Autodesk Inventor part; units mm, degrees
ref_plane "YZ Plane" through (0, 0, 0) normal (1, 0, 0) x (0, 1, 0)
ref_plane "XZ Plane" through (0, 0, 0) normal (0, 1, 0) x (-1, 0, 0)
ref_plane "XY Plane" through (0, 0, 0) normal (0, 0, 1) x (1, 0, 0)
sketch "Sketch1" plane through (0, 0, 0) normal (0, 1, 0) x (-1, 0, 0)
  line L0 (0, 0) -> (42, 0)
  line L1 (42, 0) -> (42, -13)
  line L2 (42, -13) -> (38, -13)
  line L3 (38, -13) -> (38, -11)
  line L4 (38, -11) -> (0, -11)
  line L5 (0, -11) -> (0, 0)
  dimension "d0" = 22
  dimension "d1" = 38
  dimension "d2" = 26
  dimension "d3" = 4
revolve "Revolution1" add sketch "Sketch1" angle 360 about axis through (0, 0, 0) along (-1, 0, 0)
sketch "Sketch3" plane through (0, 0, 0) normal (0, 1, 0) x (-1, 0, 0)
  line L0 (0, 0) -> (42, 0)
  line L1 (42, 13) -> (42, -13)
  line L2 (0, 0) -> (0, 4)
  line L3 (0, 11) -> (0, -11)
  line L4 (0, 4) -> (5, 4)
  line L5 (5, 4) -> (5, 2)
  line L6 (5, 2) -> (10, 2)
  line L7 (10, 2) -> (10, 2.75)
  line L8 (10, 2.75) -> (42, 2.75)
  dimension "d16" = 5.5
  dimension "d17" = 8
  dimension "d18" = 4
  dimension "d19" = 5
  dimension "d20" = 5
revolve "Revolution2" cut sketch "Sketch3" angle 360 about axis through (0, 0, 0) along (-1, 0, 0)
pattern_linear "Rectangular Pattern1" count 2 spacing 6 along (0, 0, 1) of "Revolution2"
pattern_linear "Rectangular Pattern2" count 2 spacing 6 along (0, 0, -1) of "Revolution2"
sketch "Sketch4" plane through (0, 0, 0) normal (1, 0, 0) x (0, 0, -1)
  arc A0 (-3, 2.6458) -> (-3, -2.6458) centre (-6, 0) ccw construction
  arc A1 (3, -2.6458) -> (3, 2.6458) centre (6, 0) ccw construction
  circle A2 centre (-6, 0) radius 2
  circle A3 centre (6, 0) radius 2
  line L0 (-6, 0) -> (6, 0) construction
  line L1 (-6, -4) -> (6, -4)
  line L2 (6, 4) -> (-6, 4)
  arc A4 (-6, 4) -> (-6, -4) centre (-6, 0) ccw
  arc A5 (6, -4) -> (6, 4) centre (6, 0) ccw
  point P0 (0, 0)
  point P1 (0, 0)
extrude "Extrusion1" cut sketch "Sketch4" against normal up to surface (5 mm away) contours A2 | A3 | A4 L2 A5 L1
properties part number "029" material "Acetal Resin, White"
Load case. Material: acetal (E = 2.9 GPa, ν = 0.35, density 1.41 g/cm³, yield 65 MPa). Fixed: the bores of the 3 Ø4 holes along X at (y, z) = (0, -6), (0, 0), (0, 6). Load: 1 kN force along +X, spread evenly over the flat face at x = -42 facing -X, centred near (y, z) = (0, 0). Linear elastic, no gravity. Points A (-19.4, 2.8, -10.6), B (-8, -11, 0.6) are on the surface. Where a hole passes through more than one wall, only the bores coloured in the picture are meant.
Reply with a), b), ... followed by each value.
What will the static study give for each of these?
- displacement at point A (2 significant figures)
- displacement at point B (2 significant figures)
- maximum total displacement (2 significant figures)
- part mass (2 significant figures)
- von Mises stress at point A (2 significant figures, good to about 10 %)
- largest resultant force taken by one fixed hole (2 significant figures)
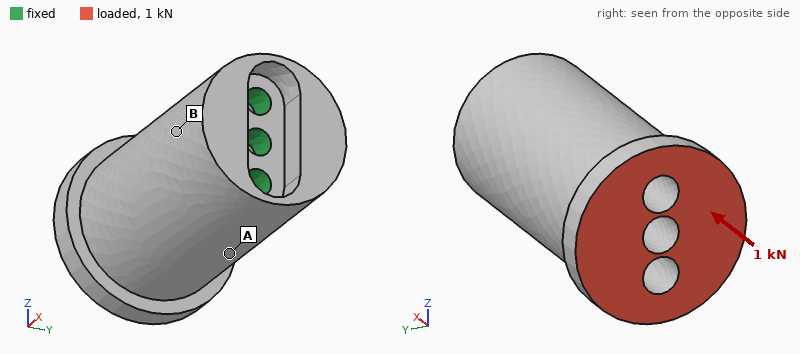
a) 26 µm
b) 24 µm
c) 59 µm
d) 19 g
e) 4.0 MPa
f) 360 N
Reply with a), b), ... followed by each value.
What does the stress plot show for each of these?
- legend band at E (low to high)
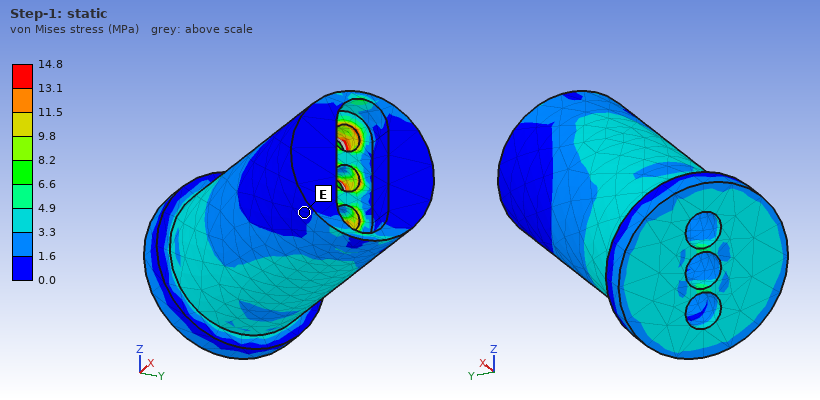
a) 0.0 to 1.6 MPa
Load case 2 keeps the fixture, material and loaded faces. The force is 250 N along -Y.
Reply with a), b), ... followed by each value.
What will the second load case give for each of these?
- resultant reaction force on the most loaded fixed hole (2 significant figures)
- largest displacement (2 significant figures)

a) 88 N
b) 0.55 mm
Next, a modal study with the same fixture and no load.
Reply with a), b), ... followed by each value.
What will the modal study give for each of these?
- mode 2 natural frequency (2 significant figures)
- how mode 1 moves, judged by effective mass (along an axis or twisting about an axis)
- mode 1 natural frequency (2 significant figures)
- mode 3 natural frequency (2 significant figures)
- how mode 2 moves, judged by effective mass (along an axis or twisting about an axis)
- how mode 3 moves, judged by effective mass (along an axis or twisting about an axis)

a) 2200 Hz
b) along Y
c) 1400 Hz
d) 4900 Hz
e) along Z
f) twisting about X
